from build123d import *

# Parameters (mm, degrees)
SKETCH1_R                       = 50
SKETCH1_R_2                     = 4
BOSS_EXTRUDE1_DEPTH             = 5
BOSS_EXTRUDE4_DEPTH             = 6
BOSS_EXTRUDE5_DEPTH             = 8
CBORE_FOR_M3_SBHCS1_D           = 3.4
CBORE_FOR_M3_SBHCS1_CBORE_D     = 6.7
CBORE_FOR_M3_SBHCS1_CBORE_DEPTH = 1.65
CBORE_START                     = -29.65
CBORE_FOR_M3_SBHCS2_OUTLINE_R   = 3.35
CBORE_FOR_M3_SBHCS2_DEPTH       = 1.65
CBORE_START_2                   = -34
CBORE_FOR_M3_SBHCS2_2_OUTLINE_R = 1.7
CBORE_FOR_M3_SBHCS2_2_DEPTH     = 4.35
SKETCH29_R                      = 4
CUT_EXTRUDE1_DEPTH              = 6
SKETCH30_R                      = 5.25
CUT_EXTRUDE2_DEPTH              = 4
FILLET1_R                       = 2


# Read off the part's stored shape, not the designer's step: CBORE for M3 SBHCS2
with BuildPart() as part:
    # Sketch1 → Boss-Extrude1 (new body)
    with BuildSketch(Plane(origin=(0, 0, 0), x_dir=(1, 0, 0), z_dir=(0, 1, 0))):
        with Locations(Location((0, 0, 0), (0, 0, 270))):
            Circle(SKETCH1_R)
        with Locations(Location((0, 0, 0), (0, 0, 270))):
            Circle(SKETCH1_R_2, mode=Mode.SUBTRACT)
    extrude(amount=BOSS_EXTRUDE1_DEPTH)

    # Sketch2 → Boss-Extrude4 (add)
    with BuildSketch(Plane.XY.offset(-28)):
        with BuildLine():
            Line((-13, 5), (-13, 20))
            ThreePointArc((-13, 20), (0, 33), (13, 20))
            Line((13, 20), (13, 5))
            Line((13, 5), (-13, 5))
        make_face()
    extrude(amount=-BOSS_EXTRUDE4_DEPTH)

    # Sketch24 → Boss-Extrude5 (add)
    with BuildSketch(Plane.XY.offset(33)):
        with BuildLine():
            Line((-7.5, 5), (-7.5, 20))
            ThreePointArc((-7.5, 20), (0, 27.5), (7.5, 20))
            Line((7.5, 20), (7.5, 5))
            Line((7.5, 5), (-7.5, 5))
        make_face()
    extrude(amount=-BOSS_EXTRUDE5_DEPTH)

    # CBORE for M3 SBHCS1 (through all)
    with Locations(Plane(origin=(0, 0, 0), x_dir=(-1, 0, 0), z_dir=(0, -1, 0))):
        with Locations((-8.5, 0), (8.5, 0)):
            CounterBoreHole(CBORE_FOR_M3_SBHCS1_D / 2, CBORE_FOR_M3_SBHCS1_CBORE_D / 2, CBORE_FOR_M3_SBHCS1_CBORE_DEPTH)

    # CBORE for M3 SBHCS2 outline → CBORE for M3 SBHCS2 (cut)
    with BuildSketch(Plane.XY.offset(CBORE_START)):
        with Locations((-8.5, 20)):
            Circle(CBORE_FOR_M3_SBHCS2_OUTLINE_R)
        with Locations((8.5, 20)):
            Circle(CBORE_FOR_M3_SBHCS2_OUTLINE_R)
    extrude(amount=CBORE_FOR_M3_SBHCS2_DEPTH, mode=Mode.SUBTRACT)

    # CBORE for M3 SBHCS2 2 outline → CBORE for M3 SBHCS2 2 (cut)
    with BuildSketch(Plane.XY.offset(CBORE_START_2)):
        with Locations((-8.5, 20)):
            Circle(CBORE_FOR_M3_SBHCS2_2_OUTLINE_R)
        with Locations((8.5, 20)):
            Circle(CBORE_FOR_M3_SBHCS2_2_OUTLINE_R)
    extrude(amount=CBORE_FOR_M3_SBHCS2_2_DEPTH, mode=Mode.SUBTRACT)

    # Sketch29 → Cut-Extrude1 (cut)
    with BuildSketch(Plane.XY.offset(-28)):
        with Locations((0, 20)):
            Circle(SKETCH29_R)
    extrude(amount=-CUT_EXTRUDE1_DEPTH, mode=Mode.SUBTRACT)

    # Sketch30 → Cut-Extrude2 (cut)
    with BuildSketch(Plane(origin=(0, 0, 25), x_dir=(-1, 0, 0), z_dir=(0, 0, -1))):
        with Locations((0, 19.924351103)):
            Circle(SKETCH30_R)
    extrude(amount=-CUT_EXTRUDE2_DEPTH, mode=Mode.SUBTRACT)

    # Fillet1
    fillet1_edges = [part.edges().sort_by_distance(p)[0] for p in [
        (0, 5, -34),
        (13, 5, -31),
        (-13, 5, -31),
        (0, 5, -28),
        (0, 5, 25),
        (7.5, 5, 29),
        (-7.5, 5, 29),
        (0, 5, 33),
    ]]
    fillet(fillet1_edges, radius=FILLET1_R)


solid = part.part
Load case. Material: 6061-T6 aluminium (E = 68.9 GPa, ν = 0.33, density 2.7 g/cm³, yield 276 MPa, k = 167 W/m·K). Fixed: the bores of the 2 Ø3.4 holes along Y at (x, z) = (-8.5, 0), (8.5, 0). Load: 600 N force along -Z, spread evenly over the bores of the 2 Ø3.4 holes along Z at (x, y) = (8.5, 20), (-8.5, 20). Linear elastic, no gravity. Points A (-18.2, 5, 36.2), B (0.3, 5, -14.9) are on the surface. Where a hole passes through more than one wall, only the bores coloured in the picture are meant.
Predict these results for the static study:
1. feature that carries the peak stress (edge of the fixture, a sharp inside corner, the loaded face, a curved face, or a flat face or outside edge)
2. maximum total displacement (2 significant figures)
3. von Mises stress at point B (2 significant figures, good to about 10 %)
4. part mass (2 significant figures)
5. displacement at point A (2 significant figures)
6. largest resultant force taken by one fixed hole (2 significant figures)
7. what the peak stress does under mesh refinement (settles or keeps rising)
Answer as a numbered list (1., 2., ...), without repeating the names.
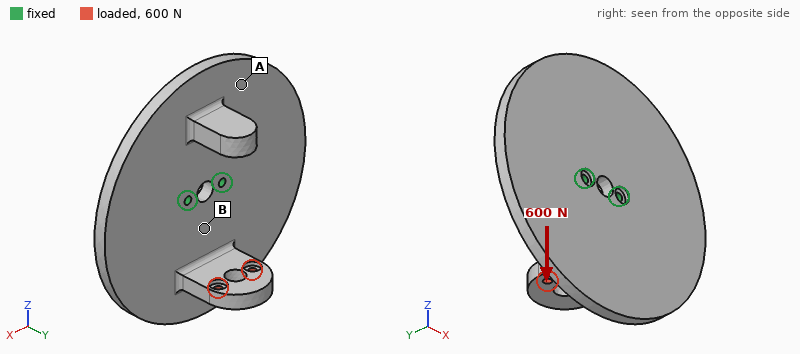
1. edge of the fixture
2. 0.37 mm
3. 36 MPa
4. 120 g
5. 0.098 mm
6. 300 N
7. keeps rising
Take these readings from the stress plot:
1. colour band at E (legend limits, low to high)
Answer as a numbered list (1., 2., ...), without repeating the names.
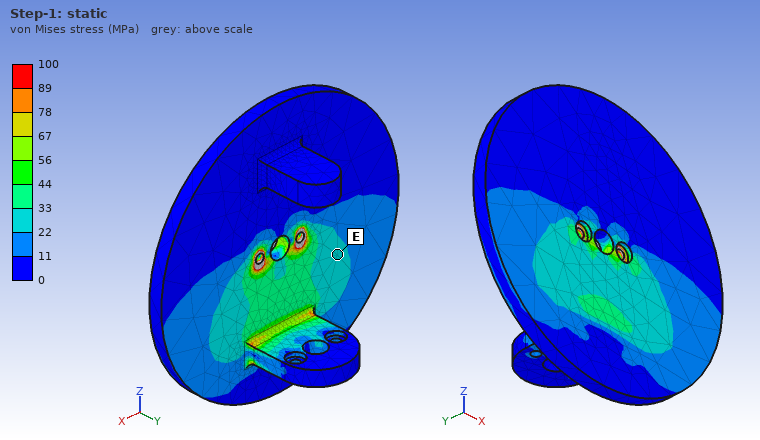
1. 22 to 33 MPa
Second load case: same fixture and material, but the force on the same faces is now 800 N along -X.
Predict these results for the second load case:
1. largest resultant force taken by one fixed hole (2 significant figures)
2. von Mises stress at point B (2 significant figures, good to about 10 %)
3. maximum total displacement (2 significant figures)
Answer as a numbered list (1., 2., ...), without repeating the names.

1. 1.5 kN
2. 47 MPa
3. 0.16 mm
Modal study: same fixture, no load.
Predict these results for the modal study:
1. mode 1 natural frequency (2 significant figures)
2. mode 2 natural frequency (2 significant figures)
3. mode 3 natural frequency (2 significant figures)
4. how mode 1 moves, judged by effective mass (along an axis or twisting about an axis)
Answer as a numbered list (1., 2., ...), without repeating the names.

1. 920 Hz
2. 1700 Hz
3. 1700 Hz
4. twisting about X
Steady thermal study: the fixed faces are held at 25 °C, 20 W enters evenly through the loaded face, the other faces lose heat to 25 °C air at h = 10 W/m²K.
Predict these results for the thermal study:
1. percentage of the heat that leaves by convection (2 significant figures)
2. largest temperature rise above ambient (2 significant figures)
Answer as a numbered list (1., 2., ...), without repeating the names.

1. 8.0 %
2. 31 K
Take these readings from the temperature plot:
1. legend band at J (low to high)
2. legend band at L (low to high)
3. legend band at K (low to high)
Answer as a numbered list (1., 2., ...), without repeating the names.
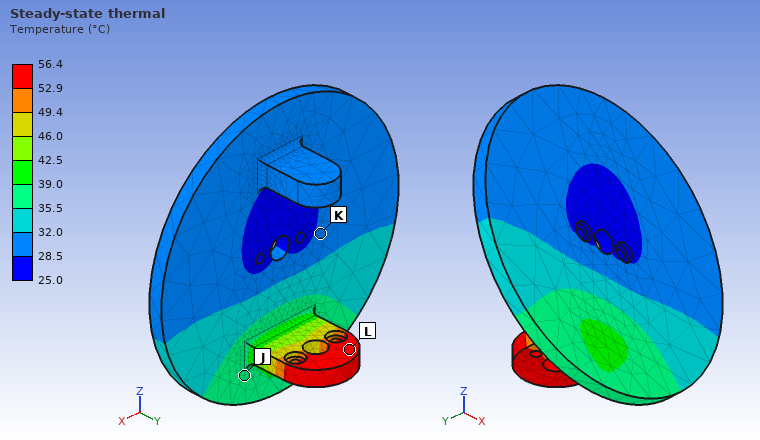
1. 35.5 to 39.0 °C
2. 52.9 to 56.4 °C
3. 28.5 to 32.0 °C
